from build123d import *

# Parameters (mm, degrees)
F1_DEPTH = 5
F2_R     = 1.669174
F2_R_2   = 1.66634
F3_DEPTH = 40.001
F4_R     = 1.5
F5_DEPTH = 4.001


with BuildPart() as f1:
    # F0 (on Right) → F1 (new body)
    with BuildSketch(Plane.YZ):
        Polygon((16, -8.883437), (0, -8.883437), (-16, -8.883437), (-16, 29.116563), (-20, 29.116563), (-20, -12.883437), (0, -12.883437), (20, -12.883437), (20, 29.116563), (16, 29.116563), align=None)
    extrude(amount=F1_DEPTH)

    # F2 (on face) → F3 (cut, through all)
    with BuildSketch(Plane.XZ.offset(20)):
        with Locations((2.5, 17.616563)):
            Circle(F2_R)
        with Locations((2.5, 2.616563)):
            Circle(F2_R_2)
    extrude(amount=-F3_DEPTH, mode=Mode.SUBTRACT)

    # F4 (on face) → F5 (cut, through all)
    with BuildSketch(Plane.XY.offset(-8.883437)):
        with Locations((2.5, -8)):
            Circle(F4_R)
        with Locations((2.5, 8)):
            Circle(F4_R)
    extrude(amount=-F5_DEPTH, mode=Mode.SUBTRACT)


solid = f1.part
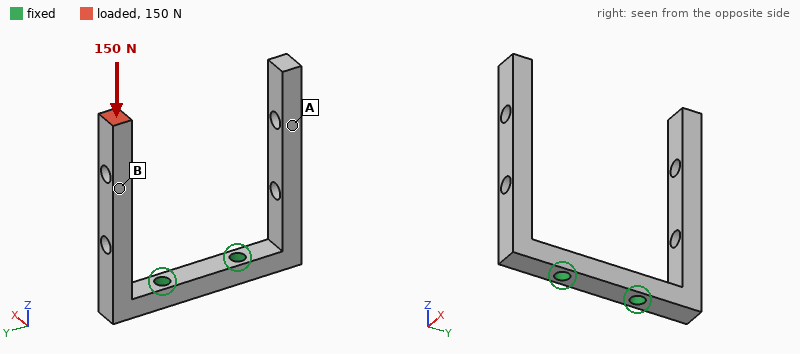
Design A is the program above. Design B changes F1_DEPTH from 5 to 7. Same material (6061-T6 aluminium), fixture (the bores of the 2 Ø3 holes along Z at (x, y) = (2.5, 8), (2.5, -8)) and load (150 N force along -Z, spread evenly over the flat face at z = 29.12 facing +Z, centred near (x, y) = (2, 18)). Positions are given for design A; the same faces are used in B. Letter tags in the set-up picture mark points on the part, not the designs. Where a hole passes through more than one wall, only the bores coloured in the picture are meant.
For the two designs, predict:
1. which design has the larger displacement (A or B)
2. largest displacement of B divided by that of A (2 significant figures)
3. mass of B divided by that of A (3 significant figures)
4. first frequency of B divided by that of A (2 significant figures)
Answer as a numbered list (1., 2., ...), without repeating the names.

1. A
2. 0.76
3. 1.44
4. 1.0
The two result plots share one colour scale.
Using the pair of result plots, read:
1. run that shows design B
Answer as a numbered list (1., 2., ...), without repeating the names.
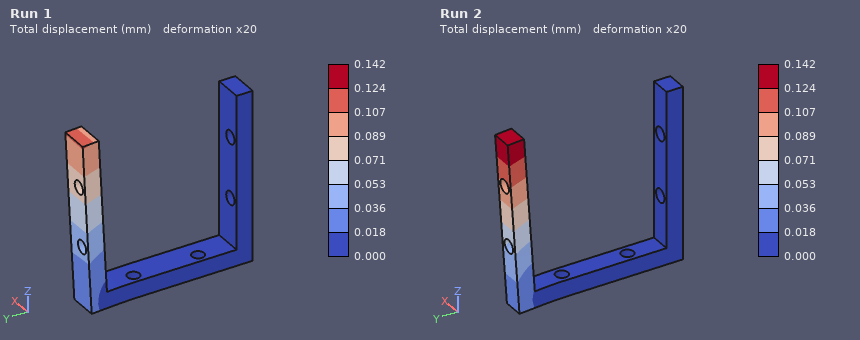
1. Run 1
